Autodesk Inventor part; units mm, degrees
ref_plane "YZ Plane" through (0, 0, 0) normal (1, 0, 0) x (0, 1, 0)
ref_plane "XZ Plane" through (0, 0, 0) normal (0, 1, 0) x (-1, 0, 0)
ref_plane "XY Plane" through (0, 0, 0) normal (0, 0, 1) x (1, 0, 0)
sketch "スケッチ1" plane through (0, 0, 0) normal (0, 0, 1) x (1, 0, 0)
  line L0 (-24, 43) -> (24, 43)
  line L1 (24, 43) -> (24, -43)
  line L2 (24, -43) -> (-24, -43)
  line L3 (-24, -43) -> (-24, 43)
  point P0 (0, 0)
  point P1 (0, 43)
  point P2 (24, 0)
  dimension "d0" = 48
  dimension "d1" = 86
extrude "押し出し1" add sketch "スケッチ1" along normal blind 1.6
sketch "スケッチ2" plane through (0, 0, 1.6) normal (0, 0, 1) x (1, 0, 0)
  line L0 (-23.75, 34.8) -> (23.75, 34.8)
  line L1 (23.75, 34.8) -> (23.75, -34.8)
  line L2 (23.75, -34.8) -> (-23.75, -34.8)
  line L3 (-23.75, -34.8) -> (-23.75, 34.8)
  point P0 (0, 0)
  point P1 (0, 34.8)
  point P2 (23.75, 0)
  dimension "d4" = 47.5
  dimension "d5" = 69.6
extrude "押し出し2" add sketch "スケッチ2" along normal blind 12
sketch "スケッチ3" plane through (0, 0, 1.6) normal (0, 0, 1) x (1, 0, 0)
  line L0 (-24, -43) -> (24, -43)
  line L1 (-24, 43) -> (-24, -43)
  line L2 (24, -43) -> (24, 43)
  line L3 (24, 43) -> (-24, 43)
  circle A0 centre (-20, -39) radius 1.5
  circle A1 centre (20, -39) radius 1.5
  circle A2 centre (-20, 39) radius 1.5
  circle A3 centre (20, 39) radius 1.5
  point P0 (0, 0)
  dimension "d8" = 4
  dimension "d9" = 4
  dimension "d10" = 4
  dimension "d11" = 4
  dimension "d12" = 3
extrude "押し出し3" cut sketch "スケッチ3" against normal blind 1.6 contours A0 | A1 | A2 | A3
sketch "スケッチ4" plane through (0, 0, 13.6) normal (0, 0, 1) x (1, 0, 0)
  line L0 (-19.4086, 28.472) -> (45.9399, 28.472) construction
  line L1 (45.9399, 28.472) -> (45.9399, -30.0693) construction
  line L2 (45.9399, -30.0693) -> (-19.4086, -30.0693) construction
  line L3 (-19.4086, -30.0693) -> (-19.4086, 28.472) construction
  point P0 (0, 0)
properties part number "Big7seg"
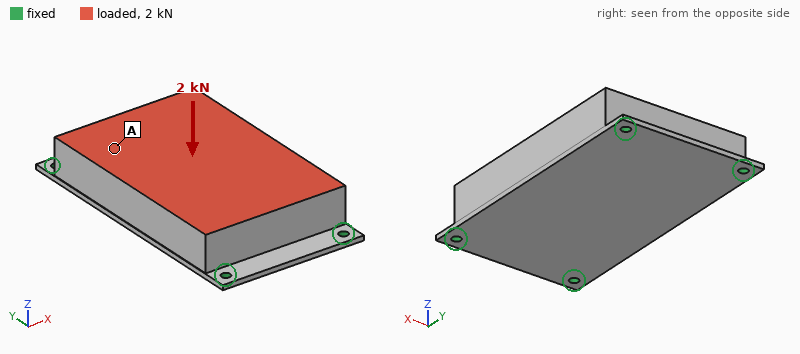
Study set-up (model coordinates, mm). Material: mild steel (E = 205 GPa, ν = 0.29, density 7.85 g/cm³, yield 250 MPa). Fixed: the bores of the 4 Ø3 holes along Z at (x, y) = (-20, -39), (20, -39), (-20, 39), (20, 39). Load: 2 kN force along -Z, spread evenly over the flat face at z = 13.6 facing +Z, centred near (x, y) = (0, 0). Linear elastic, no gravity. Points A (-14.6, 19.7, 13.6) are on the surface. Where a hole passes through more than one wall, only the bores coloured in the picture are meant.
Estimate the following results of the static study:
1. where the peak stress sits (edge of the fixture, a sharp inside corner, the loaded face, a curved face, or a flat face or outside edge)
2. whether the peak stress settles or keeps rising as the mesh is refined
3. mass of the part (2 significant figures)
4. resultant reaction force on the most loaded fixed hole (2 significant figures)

edge of the fixture
keeps rising
360 g
680 N
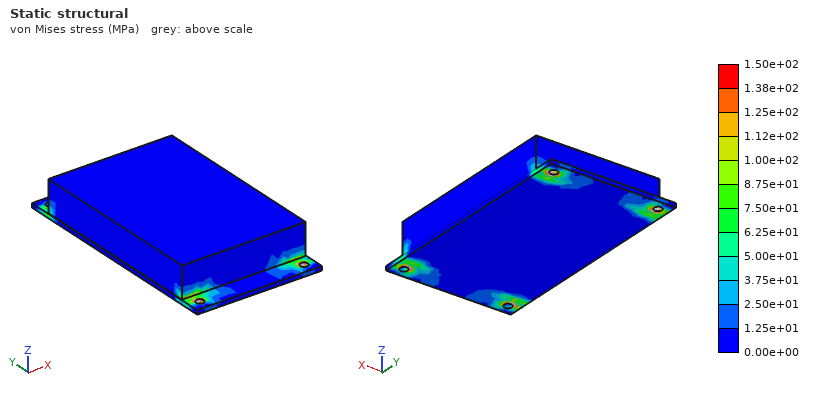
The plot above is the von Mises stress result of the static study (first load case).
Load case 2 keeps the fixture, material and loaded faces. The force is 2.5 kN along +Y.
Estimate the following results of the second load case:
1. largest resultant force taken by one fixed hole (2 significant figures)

680 N
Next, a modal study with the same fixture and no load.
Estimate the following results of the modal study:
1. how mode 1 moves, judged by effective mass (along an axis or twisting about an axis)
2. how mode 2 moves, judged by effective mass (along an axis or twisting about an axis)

along Z
along X
